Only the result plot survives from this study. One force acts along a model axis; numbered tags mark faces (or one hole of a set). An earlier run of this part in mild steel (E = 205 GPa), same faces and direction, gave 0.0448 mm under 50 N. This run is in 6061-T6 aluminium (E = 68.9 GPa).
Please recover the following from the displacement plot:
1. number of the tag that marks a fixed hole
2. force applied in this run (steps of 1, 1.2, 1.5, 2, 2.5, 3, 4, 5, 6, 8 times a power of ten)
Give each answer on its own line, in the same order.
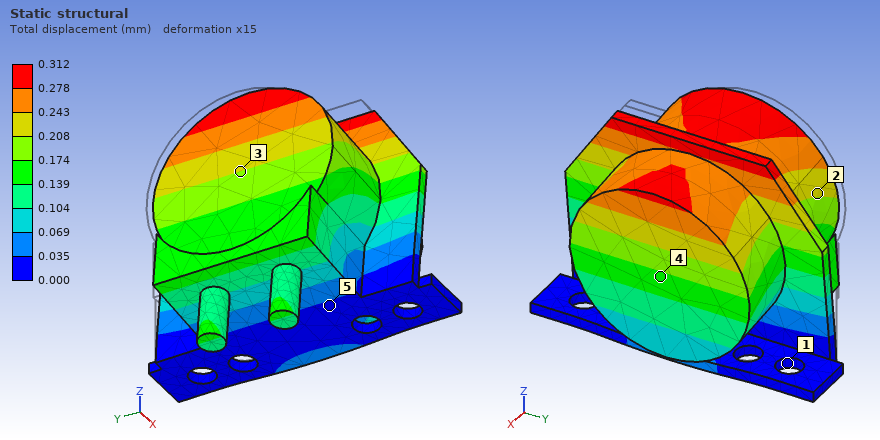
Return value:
1
120 N
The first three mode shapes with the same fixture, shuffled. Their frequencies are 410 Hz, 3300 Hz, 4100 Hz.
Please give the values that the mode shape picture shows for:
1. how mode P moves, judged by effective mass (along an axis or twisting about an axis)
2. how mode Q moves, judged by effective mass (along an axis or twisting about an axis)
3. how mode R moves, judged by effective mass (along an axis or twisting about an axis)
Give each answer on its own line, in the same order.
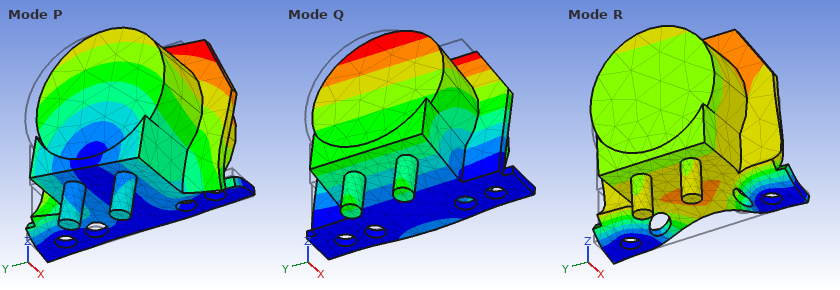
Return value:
along Y
along X
along Z
